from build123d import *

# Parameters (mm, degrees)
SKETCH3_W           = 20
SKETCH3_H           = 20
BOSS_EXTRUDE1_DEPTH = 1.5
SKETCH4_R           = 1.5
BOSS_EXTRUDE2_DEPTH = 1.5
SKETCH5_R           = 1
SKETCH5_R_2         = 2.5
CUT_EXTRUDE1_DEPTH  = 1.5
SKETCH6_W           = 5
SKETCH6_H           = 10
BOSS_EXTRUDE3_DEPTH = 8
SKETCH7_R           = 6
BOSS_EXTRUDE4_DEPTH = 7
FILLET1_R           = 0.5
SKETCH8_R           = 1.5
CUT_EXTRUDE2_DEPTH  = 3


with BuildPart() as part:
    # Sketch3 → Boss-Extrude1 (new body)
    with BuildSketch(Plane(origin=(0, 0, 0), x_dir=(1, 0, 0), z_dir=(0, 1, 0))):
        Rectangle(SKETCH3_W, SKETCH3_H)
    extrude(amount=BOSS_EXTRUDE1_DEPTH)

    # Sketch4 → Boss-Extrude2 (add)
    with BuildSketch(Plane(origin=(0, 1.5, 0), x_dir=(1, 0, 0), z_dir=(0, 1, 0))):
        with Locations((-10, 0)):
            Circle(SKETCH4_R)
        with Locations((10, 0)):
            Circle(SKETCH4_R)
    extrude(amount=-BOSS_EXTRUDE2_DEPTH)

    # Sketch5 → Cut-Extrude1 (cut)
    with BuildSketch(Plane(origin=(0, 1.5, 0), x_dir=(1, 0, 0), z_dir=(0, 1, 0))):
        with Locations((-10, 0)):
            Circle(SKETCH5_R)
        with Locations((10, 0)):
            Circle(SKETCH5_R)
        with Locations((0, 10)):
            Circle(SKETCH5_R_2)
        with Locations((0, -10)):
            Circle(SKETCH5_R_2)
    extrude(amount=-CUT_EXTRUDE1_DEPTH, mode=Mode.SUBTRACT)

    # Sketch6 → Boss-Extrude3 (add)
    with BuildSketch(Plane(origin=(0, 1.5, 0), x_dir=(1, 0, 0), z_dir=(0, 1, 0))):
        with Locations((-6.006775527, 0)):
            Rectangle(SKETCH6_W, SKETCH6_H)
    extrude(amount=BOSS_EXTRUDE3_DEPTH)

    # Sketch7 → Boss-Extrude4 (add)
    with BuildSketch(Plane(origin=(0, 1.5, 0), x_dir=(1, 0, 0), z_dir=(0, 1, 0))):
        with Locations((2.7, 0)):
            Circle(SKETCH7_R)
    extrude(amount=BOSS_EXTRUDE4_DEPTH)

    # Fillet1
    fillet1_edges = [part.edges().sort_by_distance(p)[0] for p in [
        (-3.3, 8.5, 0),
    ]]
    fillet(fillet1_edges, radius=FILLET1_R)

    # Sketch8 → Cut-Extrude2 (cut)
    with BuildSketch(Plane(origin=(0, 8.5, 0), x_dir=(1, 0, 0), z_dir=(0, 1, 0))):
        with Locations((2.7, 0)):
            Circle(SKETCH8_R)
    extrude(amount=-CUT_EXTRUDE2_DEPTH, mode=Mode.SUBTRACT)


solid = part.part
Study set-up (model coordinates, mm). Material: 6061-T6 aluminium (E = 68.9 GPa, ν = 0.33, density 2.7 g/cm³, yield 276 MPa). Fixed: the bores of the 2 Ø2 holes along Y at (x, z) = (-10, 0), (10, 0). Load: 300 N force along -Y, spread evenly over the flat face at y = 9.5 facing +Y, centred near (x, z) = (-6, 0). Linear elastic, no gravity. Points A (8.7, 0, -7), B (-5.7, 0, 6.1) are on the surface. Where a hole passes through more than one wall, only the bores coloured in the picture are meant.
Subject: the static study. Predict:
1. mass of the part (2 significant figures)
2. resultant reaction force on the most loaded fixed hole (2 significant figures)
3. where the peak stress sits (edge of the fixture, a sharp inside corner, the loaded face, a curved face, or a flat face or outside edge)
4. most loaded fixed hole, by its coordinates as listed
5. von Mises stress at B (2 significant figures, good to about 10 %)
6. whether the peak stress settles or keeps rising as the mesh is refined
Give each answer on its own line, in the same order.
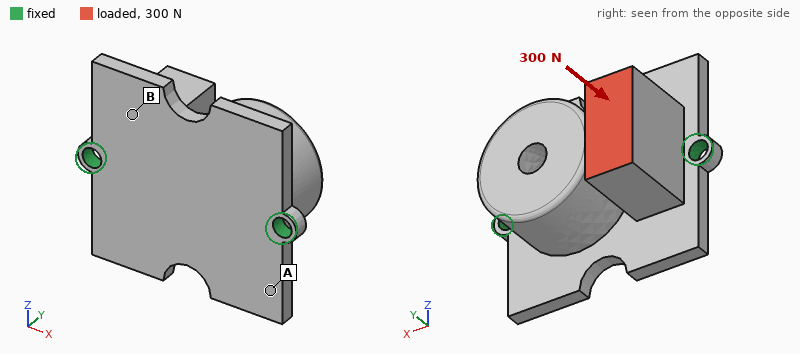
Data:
4.7 g
260 N
edge of the fixture
(-10, 0)
20 MPa
keeps rising
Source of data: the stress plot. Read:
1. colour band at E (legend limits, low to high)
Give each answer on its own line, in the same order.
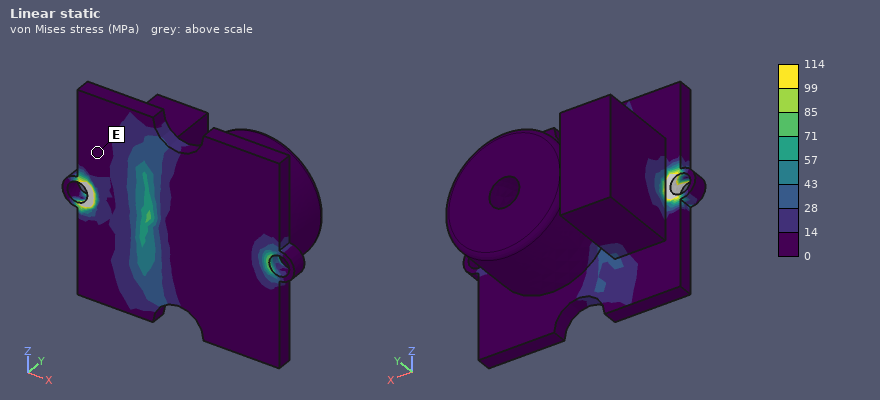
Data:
0 to 14 MPa
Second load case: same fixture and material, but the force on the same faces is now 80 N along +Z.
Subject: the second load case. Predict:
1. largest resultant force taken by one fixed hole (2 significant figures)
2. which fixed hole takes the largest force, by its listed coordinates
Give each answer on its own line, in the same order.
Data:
65 N
(-10, 0)
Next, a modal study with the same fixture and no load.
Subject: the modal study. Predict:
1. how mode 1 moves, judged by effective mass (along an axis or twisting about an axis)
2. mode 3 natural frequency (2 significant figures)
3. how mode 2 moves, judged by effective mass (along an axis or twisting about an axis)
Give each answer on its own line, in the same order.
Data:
along Z
21 kHz
along Y
